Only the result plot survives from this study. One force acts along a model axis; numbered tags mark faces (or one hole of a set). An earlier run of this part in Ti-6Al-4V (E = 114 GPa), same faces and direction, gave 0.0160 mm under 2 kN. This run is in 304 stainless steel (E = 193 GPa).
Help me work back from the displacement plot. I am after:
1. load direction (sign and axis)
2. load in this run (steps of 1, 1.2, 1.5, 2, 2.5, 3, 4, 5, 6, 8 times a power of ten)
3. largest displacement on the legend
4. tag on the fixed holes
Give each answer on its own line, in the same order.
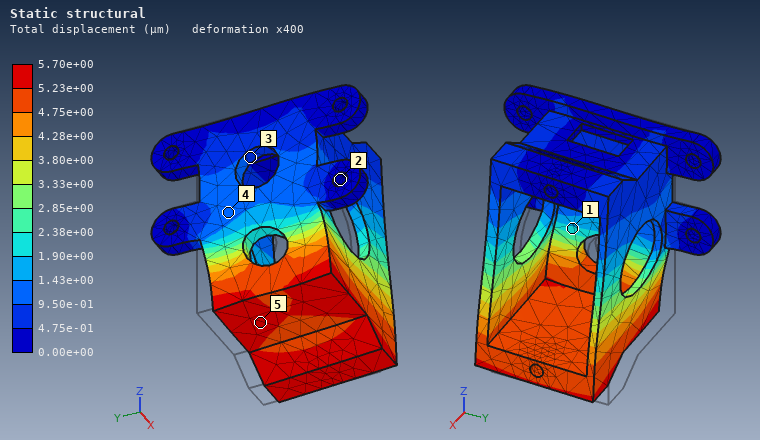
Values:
-Y
1.2 kN
5.70e+00 µm
2
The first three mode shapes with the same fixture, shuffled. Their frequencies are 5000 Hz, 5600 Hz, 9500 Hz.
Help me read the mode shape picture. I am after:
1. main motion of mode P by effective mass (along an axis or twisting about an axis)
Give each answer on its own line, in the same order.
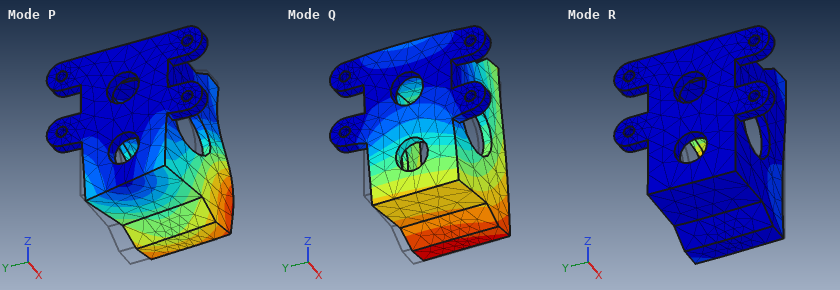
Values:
along Y
